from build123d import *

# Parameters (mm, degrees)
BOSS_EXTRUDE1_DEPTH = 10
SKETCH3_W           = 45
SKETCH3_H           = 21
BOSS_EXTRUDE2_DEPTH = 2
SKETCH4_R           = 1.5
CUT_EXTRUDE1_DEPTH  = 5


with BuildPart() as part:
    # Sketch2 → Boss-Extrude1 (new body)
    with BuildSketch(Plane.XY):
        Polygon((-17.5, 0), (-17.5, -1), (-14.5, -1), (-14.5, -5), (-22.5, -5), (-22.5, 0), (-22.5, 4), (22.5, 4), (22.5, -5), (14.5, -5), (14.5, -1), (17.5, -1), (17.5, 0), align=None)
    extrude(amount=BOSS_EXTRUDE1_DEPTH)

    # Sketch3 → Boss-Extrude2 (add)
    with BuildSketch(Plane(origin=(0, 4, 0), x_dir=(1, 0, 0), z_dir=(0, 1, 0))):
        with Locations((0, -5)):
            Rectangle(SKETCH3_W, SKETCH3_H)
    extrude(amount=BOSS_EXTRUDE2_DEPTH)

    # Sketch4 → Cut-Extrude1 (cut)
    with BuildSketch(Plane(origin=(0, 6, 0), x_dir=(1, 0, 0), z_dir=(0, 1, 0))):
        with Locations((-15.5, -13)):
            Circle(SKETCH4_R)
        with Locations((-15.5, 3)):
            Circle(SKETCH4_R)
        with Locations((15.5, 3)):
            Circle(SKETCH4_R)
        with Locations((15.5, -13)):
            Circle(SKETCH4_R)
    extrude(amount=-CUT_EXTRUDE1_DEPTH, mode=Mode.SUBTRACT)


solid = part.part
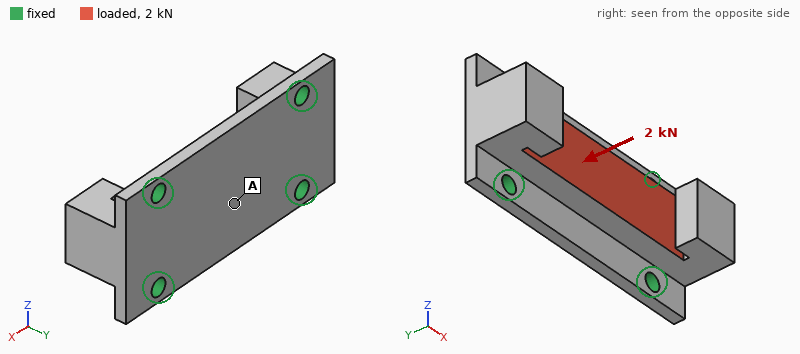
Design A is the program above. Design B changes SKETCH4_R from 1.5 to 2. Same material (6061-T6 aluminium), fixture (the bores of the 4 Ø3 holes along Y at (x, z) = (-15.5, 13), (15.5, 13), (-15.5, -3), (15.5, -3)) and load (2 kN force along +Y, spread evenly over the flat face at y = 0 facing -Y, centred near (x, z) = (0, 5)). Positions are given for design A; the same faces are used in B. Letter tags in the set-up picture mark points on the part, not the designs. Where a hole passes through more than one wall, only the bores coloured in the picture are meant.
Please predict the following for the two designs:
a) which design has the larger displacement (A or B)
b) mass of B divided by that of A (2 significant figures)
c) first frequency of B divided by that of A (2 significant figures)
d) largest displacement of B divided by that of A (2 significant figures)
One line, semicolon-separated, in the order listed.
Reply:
A; 0.99; 1.1; 0.84
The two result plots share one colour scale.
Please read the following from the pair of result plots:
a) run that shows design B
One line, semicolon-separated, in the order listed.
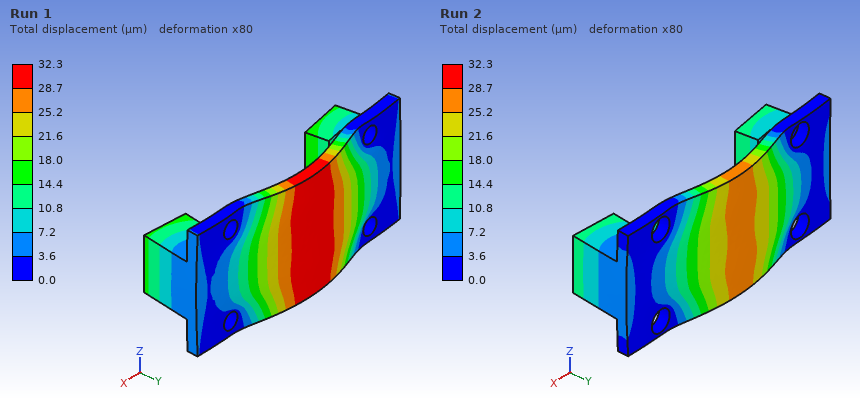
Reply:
Run 2
